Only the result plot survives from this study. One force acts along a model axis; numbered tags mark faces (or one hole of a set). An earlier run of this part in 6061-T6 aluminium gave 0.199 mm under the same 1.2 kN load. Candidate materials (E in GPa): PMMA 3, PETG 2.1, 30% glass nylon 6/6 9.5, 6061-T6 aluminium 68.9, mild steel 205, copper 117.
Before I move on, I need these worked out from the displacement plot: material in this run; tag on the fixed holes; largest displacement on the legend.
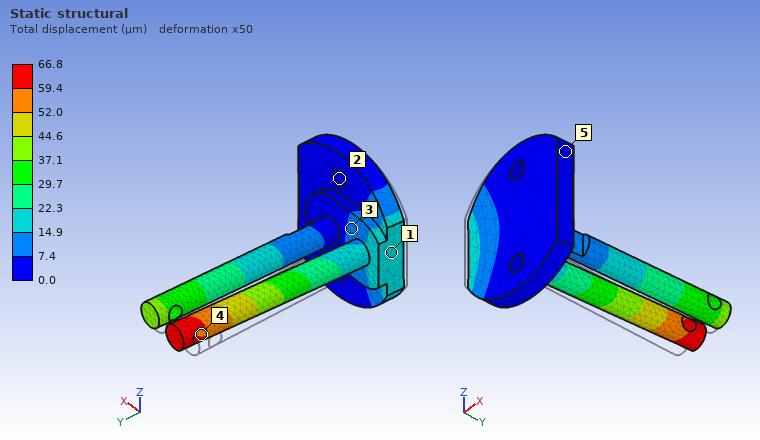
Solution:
mild steel
2
66.8 µm
